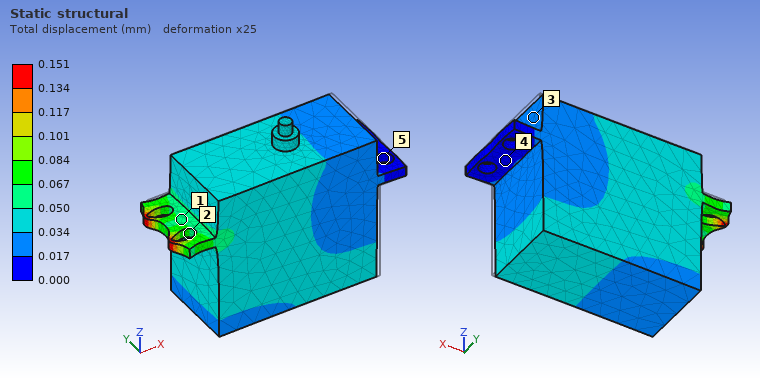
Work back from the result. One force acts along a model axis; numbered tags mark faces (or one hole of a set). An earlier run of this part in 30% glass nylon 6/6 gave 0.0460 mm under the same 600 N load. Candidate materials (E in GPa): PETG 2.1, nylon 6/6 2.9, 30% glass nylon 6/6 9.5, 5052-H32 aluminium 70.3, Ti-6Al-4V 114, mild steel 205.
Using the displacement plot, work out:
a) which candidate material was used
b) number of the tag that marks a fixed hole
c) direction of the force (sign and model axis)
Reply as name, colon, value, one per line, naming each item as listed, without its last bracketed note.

which candidate material was used: nylon 6/6
number of the tag that marks a fixed hole: 5
direction of the force: -X
